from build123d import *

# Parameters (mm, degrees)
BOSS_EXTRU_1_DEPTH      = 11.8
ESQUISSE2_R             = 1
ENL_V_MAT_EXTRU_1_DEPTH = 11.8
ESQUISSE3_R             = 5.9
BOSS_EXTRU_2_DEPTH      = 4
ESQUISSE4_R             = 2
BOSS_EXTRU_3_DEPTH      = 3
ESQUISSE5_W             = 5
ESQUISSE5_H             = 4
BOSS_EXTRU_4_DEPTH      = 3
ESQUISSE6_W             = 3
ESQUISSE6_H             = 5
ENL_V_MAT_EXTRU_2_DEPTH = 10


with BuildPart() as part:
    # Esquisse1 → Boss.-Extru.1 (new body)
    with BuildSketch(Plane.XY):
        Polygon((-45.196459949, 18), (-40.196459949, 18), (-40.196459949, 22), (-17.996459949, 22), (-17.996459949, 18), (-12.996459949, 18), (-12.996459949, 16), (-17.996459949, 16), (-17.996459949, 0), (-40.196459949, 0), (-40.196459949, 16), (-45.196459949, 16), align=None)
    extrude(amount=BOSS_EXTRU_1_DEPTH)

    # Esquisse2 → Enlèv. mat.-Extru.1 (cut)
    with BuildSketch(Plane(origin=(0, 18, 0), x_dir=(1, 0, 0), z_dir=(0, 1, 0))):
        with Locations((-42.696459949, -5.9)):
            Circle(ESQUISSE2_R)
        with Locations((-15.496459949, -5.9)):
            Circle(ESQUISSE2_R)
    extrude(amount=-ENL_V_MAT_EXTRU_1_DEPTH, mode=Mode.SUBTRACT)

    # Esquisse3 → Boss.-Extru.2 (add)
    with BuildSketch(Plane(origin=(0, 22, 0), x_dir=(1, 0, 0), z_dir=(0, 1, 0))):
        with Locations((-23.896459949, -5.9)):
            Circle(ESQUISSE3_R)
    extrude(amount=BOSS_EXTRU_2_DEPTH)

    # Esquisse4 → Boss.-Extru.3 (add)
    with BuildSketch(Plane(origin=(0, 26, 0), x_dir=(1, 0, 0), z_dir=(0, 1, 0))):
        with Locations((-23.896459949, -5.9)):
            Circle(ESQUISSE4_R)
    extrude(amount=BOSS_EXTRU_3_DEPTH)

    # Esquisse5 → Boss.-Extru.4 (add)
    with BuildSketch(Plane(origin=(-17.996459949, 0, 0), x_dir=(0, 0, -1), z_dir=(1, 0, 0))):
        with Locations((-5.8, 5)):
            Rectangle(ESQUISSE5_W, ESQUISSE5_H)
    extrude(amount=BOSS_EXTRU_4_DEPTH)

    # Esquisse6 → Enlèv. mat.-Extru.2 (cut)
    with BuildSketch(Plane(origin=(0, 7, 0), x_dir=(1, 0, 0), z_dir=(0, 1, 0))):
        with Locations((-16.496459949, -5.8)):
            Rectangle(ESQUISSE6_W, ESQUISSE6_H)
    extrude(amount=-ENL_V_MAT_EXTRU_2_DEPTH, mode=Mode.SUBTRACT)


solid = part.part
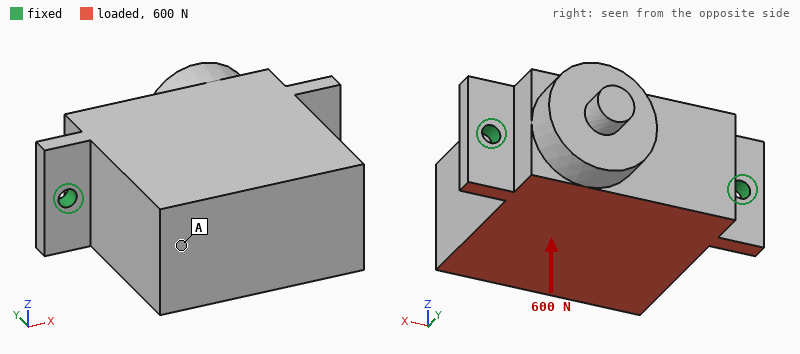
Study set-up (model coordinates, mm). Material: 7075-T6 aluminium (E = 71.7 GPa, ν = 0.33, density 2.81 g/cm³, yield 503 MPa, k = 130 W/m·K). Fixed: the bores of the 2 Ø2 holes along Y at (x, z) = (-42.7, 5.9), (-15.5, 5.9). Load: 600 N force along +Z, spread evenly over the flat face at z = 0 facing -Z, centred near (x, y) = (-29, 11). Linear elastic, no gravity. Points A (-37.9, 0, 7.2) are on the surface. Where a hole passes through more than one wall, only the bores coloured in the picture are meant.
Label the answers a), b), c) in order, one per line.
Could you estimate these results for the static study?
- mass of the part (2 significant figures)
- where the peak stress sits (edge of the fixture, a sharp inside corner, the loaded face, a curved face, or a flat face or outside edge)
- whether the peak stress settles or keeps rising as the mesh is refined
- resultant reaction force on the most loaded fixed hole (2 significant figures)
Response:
a) 18 g
b) edge of the fixture
c) keeps rising
d) 300 N
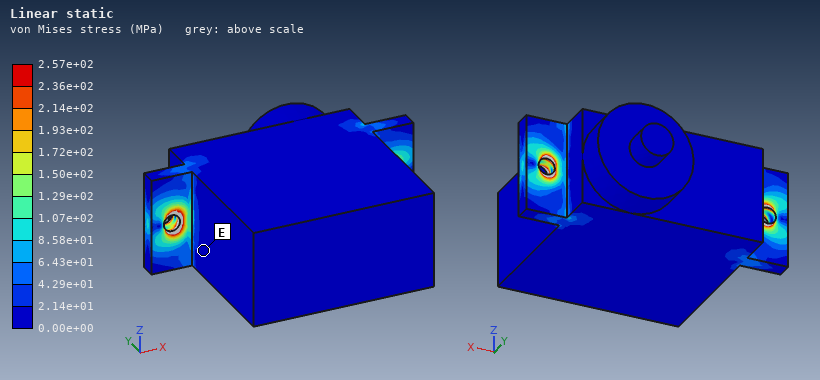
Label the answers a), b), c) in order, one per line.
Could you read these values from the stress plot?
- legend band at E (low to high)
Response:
a) 0.00e+00 to 2.14e+01 MPa
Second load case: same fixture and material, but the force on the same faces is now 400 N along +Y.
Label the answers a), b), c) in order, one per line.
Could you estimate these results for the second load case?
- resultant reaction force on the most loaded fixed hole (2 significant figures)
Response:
a) 200 N
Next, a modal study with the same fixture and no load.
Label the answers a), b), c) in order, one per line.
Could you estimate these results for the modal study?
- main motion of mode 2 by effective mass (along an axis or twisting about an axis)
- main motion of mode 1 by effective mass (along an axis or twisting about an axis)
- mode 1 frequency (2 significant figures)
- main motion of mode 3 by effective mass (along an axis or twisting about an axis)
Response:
a) along Y
b) along Z
c) 3200 Hz
d) along X
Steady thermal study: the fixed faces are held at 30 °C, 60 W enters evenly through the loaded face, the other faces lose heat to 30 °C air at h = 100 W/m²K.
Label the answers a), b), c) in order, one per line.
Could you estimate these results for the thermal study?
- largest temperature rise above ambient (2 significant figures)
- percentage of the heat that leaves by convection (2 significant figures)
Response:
a) 54 K
b) 13 %
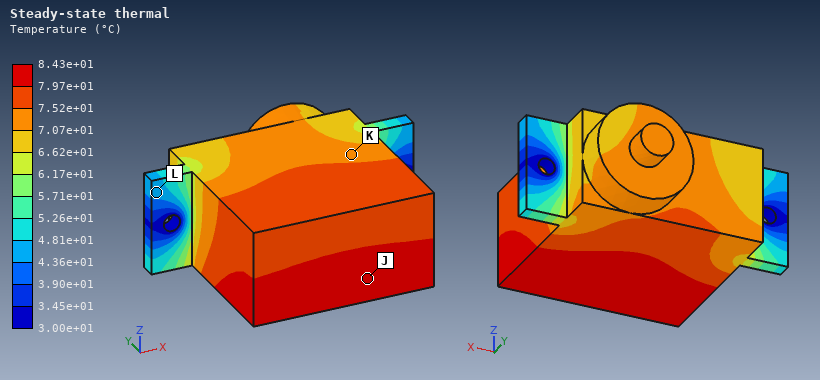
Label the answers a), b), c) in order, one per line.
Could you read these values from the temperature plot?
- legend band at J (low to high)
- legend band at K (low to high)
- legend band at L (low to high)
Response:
a) 7.97e+01 to 8.43e+01 °C
b) 7.07e+01 to 7.52e+01 °C
c) 4.36e+01 to 4.81e+01 °C
